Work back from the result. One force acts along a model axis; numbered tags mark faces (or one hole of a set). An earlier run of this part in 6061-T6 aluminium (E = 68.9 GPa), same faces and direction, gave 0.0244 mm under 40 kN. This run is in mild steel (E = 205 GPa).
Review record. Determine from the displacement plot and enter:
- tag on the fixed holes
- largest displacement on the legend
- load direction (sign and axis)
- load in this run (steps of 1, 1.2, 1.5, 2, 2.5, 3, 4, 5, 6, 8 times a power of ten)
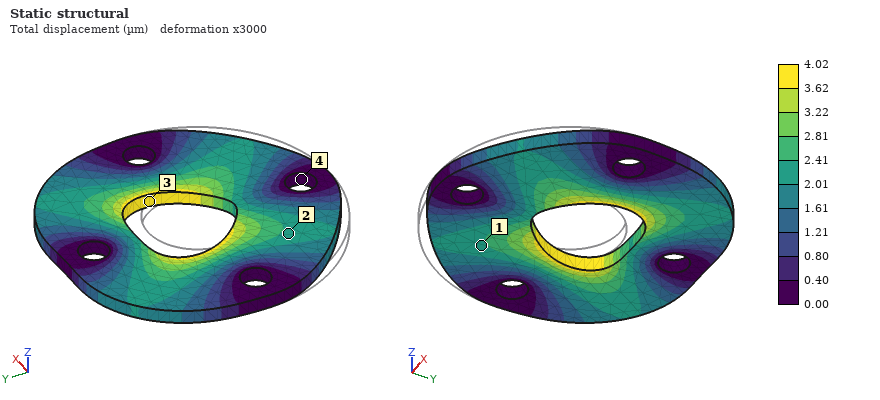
4
4.02 µm
+Y
20 kN
